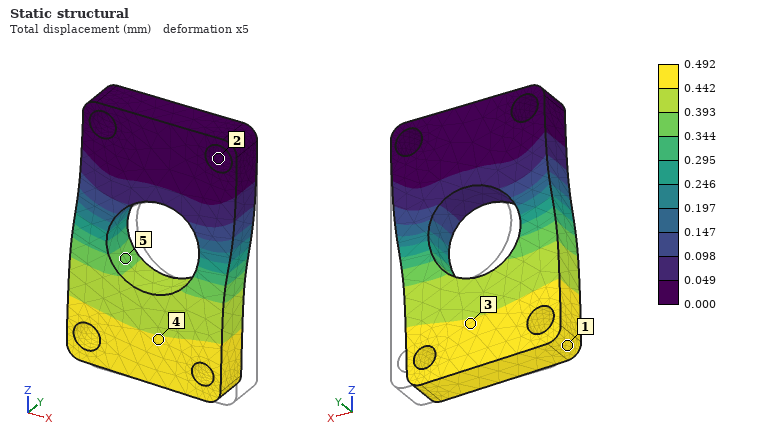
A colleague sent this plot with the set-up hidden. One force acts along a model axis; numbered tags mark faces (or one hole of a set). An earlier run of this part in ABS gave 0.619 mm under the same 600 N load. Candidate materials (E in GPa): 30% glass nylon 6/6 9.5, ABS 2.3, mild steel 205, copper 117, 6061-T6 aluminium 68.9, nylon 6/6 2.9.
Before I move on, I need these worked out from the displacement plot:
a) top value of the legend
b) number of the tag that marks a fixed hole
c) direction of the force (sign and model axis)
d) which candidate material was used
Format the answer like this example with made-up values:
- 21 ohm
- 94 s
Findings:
- 0.492 mm
- 2
- -X
- nylon 6/6
